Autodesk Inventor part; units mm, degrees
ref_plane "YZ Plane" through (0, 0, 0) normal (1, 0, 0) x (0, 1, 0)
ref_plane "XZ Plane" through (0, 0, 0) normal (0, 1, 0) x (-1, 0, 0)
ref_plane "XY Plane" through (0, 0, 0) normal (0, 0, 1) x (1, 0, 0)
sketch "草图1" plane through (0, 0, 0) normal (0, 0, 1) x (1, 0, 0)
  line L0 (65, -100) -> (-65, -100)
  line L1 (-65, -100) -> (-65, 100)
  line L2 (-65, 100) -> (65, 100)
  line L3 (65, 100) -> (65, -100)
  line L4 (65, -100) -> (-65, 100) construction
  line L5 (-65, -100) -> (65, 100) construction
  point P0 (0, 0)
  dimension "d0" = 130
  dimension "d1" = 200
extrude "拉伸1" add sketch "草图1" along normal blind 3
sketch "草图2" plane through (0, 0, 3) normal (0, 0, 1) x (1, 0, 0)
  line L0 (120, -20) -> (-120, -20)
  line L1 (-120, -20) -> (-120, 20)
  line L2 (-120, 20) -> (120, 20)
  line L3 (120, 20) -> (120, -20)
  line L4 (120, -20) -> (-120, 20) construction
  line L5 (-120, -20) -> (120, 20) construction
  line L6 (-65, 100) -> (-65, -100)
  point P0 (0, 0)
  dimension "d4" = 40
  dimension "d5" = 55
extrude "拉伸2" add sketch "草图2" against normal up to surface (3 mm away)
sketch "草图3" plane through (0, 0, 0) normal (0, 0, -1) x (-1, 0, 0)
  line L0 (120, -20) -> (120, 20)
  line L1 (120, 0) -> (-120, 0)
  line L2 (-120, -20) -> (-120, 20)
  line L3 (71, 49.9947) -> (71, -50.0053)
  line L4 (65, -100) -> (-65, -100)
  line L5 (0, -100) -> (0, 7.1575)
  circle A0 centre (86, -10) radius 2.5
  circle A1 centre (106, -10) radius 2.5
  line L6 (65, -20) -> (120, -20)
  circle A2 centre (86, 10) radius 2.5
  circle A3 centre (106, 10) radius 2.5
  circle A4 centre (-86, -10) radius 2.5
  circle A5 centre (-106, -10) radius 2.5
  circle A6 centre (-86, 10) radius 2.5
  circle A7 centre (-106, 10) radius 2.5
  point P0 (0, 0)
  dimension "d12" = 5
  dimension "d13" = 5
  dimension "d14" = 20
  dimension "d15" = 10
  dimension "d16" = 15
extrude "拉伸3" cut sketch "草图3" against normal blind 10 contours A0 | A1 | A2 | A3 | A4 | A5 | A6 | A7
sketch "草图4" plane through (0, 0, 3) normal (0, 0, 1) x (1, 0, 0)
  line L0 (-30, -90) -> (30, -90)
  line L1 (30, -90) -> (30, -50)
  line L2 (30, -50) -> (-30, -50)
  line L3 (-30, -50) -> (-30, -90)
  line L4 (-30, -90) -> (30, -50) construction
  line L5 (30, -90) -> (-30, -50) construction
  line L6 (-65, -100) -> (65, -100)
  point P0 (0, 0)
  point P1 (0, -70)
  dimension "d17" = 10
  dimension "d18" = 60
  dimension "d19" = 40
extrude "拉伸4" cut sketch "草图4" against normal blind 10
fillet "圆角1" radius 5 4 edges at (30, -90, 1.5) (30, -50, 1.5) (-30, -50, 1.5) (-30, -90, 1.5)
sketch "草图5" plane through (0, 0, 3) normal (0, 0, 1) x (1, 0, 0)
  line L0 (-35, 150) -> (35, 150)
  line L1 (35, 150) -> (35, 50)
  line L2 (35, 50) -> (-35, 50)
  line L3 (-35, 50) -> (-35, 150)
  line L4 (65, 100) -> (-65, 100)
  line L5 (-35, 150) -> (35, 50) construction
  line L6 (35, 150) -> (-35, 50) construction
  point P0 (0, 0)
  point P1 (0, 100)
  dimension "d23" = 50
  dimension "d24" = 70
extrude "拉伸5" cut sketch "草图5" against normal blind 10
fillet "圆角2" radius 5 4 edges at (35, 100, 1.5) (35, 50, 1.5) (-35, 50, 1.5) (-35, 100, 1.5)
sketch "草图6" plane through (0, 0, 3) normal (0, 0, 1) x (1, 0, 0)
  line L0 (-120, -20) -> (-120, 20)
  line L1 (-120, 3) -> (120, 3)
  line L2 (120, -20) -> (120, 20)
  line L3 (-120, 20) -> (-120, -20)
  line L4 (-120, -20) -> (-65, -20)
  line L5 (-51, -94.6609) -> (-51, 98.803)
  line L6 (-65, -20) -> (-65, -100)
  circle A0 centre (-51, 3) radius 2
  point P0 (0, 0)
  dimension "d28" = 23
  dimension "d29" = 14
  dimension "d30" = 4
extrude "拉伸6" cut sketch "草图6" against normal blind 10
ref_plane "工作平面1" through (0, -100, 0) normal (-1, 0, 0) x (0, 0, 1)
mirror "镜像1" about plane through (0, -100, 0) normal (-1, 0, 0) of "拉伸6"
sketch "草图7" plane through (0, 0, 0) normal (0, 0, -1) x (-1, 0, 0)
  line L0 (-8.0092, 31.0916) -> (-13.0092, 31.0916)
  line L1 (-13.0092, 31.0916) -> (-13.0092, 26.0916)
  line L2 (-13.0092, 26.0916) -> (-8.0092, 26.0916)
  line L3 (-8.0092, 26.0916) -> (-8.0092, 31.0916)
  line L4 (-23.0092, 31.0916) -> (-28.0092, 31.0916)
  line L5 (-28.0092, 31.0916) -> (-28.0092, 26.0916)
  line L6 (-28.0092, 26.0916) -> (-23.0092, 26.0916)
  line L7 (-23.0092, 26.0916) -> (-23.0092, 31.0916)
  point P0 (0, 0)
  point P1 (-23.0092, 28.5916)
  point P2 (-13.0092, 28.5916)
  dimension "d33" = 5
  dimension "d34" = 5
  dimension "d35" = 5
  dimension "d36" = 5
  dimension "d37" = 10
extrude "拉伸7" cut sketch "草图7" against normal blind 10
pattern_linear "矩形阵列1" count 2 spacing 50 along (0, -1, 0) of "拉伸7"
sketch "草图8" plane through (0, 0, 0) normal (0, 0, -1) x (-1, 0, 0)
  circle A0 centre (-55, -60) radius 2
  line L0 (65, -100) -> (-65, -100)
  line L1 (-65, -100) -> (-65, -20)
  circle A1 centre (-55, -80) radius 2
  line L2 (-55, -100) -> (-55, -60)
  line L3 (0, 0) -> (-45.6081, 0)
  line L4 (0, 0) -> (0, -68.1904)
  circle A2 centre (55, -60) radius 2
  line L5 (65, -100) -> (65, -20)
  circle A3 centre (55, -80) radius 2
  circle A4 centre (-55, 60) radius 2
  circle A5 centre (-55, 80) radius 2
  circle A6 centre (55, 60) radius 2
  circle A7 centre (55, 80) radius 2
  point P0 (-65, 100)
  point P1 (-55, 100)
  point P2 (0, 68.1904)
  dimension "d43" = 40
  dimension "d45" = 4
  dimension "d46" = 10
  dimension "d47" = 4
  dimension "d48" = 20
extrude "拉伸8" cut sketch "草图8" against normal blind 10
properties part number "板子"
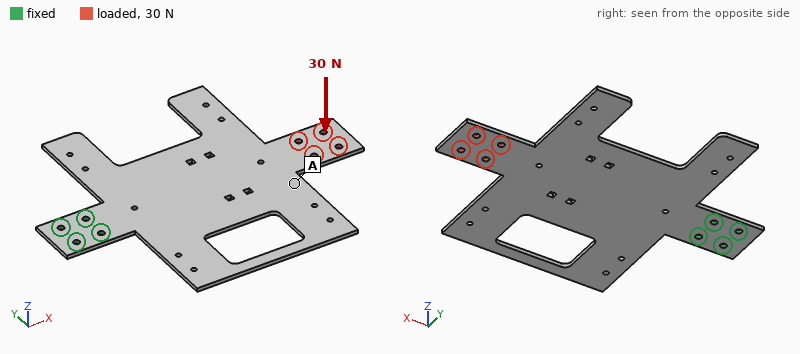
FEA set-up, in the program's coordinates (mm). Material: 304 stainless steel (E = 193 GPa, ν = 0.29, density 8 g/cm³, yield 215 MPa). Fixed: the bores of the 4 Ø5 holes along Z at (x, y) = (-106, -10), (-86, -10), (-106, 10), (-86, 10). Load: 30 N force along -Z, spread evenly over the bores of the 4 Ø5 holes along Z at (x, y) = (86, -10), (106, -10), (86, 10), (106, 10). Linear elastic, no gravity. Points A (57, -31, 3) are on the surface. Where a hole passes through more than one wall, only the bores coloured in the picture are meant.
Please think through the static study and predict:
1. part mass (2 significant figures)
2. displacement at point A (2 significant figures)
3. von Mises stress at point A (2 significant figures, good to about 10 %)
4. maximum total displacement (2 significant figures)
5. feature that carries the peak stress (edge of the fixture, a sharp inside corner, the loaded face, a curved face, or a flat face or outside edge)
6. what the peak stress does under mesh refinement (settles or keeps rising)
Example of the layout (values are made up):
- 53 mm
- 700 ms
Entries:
- 580 g
- 1.5 mm
- 12 MPa
- 2.5 mm
- edge of the fixture
- keeps rising
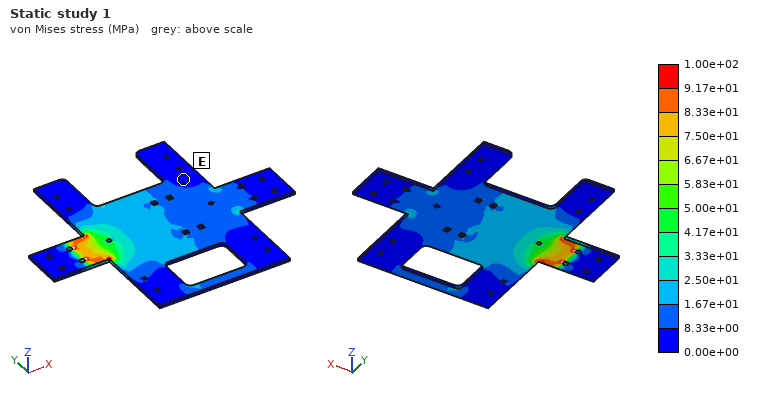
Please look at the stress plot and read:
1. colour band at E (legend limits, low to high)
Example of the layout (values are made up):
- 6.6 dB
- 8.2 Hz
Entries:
- 0.00e+00 to 8.33e+00 MPa
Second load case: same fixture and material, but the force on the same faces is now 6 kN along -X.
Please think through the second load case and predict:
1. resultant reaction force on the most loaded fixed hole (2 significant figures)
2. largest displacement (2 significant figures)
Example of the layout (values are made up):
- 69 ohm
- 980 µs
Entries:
- 2.6 kN
- 37 µm
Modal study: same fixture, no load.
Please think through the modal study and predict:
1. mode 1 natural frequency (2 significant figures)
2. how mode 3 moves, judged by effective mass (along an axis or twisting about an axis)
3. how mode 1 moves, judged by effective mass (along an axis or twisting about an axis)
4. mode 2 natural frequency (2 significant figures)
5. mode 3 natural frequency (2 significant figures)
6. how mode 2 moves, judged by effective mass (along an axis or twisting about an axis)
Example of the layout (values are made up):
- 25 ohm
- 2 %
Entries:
- 51 Hz
- along Z
- along Z
- 110 Hz
- 270 Hz
- twisting about X
